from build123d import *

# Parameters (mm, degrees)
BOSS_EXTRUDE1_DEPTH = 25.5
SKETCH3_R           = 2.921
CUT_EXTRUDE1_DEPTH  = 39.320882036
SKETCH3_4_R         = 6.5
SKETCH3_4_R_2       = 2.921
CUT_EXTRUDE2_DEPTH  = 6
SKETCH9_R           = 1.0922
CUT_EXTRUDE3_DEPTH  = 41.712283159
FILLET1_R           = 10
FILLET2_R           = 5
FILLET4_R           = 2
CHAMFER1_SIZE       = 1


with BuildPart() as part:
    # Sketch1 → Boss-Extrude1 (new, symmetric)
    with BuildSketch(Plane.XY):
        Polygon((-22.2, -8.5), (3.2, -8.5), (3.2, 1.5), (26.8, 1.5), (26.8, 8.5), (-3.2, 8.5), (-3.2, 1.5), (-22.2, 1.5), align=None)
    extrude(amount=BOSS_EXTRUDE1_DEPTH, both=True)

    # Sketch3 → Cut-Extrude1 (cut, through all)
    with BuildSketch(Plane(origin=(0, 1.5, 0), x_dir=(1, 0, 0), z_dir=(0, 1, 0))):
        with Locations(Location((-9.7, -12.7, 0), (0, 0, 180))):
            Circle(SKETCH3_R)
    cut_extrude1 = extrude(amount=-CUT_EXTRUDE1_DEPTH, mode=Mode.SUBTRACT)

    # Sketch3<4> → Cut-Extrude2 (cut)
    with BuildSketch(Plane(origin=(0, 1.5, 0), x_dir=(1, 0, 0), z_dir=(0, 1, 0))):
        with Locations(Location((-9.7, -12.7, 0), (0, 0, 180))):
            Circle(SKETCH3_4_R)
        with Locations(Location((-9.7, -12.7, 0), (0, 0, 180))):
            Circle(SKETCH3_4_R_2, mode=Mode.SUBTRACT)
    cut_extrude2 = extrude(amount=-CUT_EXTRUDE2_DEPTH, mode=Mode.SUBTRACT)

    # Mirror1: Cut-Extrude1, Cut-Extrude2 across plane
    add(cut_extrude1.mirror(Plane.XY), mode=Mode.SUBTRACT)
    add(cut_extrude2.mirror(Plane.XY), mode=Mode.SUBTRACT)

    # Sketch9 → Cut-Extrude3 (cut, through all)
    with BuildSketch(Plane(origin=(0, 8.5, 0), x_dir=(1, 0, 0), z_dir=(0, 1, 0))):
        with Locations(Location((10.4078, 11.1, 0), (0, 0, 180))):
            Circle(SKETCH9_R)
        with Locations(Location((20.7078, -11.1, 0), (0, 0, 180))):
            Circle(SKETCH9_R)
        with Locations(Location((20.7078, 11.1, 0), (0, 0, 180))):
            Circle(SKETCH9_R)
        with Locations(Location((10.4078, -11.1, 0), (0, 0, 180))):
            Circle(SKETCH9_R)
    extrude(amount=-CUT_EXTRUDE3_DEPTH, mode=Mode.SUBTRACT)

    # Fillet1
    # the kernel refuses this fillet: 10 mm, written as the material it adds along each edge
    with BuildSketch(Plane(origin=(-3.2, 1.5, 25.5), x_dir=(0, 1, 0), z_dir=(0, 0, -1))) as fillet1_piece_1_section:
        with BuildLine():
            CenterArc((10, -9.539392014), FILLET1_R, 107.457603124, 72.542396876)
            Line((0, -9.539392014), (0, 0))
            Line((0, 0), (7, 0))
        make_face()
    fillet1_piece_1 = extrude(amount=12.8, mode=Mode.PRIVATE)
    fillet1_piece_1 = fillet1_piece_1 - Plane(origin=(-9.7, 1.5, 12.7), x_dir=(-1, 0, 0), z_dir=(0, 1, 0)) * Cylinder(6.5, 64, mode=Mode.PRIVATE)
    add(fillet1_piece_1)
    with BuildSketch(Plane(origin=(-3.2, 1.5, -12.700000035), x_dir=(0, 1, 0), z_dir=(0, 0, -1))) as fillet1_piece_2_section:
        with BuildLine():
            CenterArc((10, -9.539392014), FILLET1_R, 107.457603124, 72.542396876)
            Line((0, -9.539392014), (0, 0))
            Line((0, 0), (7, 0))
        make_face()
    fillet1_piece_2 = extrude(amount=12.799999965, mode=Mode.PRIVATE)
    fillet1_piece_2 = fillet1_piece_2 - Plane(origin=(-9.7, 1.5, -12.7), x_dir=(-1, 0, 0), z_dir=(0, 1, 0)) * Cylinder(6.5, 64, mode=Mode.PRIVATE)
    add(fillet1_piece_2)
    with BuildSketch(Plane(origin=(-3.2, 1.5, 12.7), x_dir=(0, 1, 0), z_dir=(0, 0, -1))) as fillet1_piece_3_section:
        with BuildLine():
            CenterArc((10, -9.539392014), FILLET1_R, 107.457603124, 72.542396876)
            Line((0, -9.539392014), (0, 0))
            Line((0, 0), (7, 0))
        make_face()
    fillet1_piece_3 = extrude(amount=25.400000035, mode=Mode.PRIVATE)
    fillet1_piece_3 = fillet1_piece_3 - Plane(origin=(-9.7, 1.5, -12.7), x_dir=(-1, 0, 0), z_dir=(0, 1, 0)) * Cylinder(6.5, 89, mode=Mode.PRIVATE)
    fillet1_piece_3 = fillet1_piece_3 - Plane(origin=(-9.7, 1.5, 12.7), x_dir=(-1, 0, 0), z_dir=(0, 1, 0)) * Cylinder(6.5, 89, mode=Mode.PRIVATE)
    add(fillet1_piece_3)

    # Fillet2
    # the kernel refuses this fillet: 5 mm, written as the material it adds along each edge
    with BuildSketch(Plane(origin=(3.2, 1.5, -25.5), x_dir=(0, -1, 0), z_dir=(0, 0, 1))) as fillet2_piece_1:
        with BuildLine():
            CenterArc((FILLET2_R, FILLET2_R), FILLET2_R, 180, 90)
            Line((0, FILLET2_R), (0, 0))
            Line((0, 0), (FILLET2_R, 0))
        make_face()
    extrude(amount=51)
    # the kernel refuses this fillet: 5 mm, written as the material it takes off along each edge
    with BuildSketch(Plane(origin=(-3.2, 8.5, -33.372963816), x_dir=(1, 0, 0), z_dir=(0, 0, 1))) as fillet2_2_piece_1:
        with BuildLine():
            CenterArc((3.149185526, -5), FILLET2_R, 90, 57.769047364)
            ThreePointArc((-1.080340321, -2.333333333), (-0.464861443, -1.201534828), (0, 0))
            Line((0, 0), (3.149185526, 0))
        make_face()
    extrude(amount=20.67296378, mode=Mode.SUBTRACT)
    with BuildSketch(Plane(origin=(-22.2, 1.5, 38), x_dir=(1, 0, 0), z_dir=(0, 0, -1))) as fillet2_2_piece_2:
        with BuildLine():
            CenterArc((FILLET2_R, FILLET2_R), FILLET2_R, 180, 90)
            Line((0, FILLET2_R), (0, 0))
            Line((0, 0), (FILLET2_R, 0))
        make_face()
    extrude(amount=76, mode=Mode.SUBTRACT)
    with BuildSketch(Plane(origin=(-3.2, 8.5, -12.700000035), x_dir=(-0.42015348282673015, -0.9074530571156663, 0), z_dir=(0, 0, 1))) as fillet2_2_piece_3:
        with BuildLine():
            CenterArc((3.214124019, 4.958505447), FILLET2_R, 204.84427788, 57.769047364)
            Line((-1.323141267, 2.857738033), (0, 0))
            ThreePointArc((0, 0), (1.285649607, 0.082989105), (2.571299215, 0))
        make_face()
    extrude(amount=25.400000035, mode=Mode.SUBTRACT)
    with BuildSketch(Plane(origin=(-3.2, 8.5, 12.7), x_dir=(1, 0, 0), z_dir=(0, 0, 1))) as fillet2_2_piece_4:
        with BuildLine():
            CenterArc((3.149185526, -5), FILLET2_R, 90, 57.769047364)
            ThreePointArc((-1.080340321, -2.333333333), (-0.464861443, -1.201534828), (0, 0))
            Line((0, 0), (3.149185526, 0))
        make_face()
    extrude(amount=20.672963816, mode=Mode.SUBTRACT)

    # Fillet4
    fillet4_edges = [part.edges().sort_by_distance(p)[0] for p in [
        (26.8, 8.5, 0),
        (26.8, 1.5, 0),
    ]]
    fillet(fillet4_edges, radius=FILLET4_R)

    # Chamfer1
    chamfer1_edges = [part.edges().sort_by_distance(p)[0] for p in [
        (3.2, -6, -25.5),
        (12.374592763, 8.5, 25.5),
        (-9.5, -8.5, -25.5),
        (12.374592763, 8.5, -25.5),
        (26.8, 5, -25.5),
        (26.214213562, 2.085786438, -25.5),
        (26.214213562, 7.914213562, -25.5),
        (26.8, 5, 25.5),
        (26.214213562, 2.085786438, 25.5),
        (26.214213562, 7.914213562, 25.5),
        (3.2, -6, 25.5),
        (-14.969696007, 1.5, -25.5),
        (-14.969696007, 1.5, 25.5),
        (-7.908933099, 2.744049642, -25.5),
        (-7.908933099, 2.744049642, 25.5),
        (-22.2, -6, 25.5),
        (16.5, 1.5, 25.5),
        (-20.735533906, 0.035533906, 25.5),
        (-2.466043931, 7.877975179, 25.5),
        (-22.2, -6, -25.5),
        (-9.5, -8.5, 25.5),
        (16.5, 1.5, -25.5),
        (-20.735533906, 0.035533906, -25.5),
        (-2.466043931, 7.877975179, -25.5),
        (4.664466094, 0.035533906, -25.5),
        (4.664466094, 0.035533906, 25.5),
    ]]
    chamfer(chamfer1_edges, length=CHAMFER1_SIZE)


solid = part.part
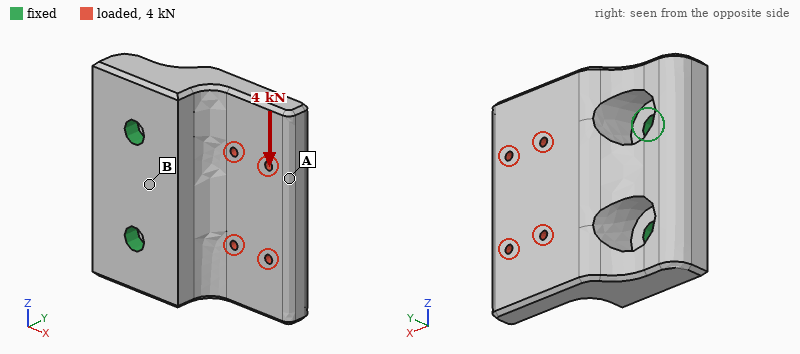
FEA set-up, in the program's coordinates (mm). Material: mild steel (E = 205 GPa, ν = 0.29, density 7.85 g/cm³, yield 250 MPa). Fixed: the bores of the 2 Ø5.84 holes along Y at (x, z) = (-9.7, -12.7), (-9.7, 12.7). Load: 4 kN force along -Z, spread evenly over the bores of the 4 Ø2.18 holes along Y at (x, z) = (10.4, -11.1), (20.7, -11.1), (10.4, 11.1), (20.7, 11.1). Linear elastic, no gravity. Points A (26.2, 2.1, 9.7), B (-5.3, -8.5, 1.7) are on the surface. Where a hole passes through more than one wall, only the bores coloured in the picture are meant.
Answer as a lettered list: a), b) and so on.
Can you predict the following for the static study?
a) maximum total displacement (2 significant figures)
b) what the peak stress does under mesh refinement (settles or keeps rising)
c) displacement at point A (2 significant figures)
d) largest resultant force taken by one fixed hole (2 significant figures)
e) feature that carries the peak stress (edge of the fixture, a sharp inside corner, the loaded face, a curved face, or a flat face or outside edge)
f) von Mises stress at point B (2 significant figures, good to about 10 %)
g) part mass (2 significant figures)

a) 19 µm
b) keeps rising
c) 16 µm
d) 4.2 kN
e) edge of the fixture
f) 35 MPa
g) 170 g
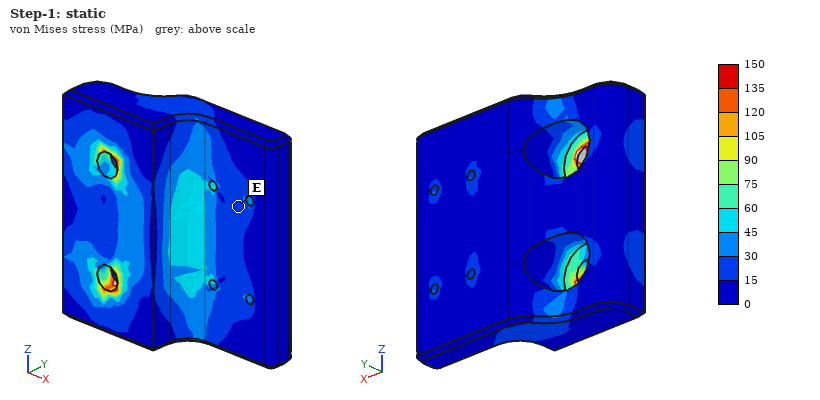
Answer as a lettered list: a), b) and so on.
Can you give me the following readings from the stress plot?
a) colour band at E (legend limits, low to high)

a) 15 to 30 MPa
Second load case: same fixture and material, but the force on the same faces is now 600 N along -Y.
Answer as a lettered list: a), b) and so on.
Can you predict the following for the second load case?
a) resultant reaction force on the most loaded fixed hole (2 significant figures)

a) 320 N
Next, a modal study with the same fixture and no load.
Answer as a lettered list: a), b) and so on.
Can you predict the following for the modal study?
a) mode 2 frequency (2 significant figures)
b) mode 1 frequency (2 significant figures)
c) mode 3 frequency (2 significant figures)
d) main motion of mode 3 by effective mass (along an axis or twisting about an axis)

a) 7700 Hz
b) 3500 Hz
c) 10 kHz
d) along Z
